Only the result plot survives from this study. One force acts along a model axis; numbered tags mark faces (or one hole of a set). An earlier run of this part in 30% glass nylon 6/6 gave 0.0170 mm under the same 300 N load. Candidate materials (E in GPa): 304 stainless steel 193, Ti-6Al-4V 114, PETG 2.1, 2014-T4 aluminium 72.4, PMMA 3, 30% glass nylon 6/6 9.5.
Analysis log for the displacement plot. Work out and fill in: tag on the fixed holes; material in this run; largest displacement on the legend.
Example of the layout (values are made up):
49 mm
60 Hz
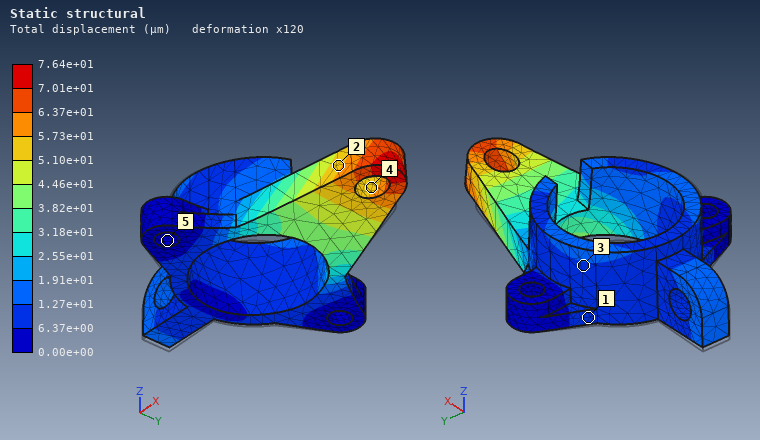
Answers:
5
PETG
7.64e+01 µm
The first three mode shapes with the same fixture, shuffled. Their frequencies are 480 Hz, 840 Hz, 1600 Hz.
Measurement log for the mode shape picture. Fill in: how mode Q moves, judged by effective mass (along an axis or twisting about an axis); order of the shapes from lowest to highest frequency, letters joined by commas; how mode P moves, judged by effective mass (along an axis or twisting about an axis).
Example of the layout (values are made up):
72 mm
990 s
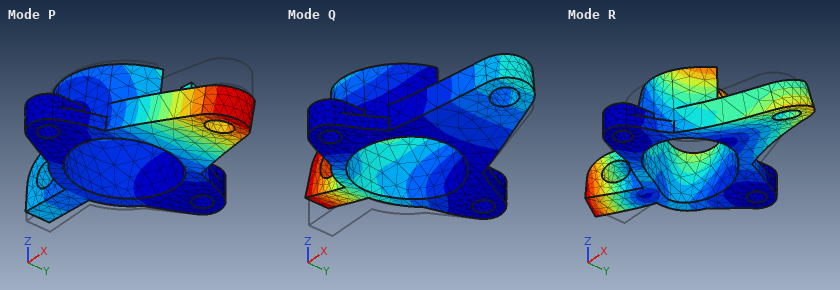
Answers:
along Z
P, Q, R
along Z
